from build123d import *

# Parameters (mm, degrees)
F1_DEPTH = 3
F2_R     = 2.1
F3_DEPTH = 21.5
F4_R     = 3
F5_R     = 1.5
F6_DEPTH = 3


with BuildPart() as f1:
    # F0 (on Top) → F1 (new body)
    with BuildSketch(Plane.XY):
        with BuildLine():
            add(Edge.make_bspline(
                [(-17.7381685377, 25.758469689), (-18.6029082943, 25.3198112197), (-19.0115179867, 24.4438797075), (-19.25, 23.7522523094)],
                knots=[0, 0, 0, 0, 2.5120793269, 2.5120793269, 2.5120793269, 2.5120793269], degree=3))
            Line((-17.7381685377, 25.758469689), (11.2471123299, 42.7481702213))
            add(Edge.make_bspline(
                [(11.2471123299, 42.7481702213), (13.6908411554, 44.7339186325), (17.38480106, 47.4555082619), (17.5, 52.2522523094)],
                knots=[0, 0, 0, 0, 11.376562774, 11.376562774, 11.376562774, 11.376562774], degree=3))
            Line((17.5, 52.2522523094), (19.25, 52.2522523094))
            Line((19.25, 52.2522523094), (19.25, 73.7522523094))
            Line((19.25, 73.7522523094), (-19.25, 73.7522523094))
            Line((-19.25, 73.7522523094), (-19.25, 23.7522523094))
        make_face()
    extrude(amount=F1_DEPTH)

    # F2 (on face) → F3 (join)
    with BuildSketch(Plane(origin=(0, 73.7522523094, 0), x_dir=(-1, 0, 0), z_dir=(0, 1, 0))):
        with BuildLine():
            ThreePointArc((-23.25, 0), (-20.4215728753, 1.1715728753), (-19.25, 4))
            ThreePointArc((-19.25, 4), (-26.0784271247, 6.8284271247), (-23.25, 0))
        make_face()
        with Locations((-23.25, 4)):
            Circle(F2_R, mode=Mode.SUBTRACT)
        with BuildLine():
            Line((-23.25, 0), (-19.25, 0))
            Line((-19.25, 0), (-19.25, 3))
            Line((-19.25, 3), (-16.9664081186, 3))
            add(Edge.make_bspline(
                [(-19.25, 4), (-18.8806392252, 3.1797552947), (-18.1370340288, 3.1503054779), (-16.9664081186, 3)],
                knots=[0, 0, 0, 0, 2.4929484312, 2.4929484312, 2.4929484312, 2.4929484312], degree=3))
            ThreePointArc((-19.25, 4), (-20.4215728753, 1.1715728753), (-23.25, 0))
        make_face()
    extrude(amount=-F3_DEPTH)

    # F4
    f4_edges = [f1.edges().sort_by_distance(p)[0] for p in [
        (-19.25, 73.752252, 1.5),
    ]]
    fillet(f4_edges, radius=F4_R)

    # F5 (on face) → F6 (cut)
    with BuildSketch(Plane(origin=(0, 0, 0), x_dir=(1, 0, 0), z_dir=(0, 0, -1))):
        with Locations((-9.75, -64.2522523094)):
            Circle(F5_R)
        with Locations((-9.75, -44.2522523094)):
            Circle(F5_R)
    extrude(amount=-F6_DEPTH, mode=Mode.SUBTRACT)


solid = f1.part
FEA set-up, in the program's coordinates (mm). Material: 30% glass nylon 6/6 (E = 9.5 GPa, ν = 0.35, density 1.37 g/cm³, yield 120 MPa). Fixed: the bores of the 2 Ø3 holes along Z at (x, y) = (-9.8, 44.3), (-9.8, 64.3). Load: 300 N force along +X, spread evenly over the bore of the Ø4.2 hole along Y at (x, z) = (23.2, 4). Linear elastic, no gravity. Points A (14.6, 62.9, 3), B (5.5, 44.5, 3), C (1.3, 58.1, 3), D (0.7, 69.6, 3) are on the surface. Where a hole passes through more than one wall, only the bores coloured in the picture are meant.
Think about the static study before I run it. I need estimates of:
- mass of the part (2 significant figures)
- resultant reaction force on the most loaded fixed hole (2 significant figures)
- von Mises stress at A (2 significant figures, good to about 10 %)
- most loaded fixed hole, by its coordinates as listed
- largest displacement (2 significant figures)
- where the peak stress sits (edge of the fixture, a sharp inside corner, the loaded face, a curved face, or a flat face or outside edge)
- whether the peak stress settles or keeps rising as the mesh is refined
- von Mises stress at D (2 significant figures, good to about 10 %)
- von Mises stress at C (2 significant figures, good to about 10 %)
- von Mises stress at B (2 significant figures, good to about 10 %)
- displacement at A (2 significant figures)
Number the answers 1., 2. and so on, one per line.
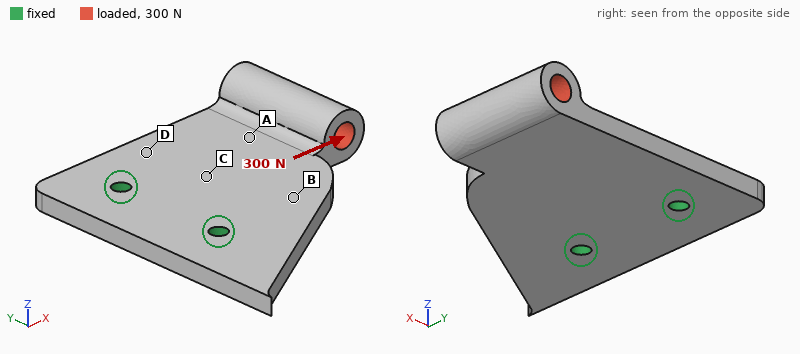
1. 7.0 g
2. 270 N
3. 23 MPa
4. (-9.8, 64.3)
5. 0.76 mm
6. edge of the fixture
7. keeps rising
8. 20 MPa
9. 17 MPa
10. 13 MPa
11. 0.32 mm
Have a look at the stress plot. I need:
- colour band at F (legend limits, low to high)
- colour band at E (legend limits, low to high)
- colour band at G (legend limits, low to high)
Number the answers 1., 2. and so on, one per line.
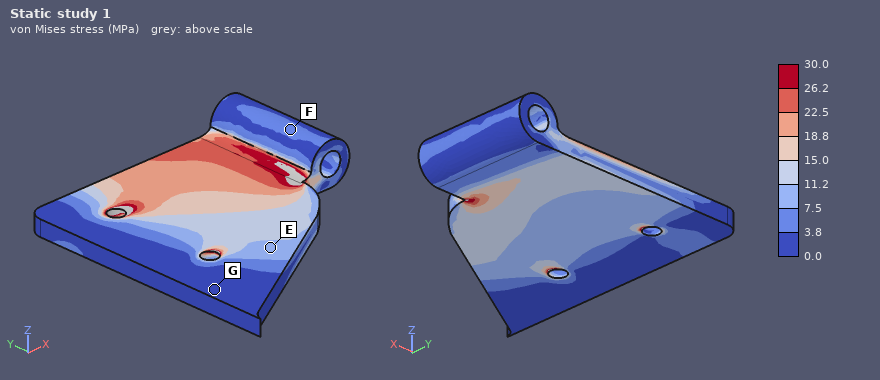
1. 3.8 to 7.5 MPa
2. 7.5 to 11.2 MPa
3. 0.0 to 3.8 MPa
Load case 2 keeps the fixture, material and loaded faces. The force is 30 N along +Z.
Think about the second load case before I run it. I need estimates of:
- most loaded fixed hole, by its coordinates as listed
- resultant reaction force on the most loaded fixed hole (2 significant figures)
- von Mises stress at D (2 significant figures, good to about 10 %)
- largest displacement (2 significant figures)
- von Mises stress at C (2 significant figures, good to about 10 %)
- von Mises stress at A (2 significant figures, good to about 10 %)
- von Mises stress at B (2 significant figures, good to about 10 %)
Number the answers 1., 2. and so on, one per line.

1. (-9.8, 64.3)
2. 26 N
3. 13 MPa
4. 0.66 mm
5. 12 MPa
6. 6.7 MPa
7. 11 MPa
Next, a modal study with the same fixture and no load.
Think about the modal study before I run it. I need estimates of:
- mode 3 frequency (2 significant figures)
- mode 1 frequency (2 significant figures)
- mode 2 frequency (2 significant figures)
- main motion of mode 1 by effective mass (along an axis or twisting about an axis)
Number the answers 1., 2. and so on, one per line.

1. 4900 Hz
2. 930 Hz
3. 3000 Hz
4. along Z
